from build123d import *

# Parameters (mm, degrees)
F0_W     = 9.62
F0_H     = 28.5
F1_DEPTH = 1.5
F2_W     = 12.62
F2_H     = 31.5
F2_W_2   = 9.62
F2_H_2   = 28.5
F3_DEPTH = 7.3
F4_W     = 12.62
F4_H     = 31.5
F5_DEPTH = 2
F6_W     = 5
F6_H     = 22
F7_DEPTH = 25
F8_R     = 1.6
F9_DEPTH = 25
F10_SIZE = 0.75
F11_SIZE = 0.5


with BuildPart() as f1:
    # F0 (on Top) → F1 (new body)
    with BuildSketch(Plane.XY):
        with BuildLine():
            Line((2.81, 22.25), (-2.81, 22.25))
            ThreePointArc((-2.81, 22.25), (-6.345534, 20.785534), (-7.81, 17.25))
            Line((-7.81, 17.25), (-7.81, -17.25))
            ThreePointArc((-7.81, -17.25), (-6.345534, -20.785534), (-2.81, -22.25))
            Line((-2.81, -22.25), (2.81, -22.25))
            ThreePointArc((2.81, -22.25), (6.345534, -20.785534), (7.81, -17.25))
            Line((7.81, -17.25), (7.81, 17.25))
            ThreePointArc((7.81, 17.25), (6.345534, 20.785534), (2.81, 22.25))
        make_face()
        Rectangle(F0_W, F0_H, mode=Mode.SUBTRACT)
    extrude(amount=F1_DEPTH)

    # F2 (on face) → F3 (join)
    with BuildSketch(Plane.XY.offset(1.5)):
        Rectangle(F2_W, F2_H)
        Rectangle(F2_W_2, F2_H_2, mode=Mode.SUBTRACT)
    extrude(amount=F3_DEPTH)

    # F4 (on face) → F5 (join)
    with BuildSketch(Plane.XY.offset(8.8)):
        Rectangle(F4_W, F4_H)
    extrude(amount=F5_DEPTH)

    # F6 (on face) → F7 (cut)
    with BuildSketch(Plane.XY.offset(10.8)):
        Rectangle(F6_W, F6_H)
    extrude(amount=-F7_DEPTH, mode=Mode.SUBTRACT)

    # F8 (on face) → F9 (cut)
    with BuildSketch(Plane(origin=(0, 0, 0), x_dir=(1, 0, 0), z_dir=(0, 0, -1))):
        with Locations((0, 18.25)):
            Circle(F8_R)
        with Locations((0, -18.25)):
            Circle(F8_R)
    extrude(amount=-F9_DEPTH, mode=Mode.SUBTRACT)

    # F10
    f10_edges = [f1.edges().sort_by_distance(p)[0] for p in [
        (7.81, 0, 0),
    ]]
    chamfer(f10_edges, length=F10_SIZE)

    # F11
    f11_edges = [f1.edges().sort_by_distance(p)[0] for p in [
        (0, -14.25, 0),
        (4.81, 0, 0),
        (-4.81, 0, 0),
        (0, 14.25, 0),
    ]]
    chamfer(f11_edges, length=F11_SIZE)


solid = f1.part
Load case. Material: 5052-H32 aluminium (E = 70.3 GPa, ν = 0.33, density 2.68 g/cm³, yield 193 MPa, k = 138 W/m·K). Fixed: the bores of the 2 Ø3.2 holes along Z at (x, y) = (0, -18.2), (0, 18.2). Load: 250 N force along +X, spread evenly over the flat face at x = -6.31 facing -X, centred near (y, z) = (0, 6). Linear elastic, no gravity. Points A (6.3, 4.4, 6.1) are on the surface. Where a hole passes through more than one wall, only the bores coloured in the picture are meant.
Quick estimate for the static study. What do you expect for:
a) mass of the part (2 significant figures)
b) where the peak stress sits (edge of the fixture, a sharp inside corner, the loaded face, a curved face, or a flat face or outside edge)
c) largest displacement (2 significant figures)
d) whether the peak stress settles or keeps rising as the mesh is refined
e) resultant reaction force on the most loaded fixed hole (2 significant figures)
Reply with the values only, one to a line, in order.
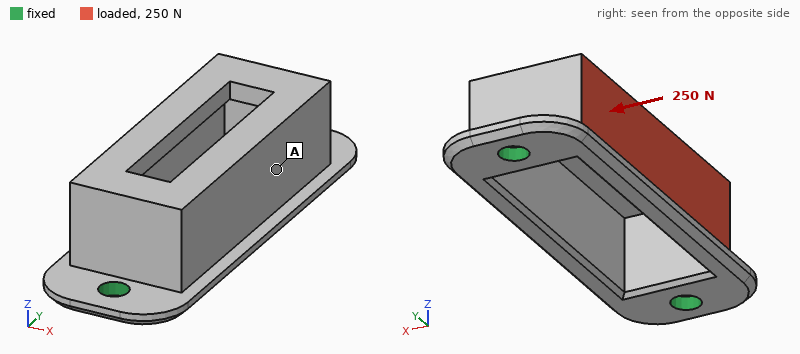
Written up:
5.4 g
edge of the fixture
41 µm
keeps rising
130 N
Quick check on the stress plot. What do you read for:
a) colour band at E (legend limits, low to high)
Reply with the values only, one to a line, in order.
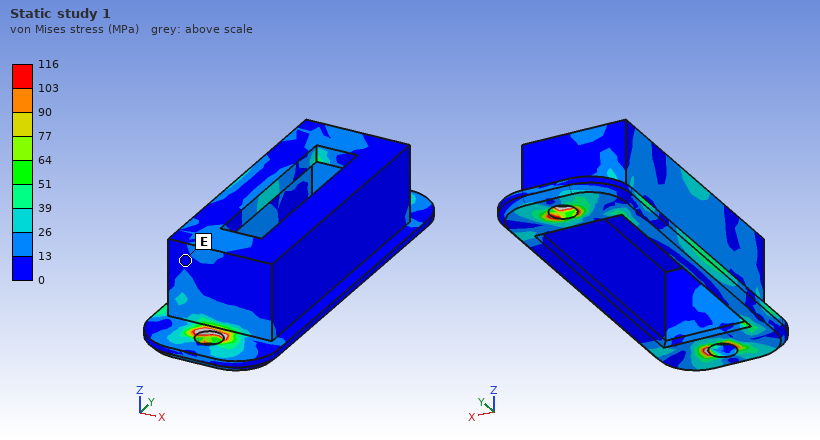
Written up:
0 to 13 MPa
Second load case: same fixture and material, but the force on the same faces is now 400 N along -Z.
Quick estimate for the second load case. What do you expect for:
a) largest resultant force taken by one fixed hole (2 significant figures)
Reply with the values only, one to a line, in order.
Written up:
230 N
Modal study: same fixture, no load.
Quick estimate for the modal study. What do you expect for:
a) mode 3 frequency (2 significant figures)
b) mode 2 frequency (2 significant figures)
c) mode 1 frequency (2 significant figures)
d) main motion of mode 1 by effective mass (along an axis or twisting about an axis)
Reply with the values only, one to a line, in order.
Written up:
14 kHz
14 kHz
6400 Hz
along X
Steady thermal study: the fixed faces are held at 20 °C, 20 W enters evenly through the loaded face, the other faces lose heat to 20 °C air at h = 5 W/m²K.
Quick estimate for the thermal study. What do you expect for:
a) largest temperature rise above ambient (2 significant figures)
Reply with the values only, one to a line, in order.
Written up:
49 K
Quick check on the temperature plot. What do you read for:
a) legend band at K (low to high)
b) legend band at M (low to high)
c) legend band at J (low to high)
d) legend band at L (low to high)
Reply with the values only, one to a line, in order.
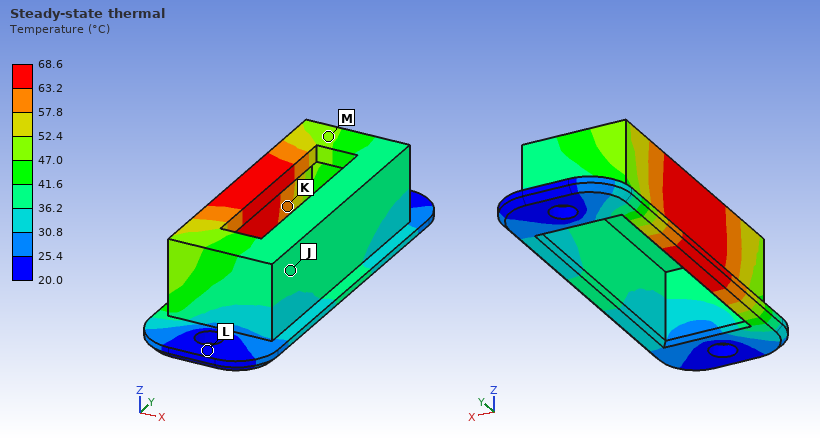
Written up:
57.8 to 63.2 °C
47.0 to 52.4 °C
36.2 to 41.6 °C
20.0 to 25.4 °C
